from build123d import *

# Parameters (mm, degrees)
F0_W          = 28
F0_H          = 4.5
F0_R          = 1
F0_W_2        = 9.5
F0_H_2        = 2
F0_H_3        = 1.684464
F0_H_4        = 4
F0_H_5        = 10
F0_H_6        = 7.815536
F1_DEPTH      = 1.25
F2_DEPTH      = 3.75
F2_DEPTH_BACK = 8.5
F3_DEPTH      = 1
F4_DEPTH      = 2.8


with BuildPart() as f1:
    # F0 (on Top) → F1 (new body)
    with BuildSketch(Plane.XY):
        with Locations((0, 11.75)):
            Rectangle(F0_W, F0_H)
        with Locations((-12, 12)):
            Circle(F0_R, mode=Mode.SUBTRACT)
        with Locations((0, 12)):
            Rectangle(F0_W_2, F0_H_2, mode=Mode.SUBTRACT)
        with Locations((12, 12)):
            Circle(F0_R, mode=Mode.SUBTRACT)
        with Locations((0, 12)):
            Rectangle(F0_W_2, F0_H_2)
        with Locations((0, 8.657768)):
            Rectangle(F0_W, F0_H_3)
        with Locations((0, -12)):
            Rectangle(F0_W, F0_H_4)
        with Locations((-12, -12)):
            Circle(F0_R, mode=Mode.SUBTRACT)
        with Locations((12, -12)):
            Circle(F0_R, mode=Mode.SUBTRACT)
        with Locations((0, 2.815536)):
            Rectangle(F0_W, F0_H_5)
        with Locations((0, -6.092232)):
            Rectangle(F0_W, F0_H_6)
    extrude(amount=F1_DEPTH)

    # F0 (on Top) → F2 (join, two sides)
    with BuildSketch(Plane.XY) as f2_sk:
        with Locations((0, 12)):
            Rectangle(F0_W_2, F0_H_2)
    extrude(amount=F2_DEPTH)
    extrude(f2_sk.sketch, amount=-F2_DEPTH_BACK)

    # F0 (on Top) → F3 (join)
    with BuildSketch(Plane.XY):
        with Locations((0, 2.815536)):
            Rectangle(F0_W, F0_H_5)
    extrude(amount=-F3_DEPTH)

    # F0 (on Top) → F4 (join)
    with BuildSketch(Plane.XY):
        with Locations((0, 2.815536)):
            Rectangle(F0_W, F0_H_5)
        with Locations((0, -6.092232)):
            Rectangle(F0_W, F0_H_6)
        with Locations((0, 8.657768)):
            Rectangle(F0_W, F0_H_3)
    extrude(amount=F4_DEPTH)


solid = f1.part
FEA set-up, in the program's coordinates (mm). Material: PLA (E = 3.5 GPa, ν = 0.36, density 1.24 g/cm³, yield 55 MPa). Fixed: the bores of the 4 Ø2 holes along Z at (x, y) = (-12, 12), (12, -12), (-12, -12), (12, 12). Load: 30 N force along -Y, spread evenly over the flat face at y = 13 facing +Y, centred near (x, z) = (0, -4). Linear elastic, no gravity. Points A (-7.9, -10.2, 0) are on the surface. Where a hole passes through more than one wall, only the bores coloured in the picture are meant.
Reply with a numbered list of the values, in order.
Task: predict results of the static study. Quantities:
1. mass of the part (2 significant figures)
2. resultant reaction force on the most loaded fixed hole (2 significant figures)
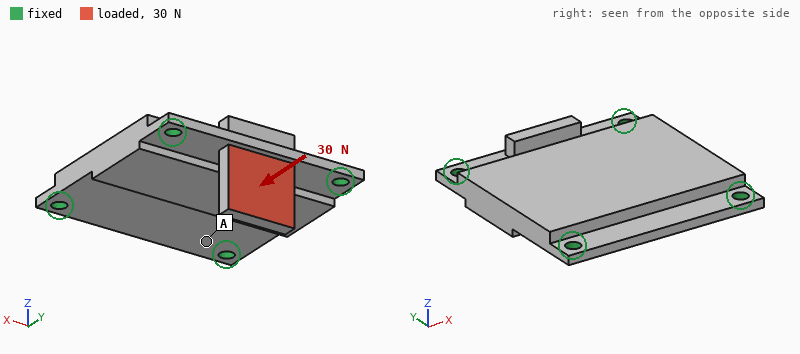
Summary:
1. 2.9 g
2. 12 N
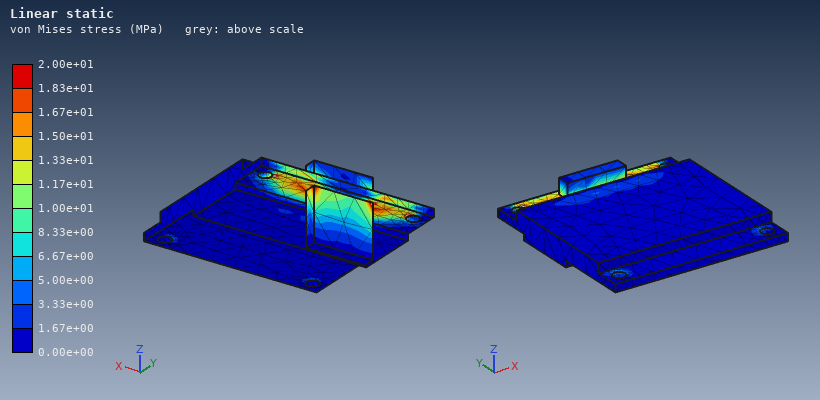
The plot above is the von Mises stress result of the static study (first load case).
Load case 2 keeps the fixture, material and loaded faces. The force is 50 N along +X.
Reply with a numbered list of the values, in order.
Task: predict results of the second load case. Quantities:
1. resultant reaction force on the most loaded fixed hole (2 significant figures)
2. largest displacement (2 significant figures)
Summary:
1. 24 N
2. 0.11 mm
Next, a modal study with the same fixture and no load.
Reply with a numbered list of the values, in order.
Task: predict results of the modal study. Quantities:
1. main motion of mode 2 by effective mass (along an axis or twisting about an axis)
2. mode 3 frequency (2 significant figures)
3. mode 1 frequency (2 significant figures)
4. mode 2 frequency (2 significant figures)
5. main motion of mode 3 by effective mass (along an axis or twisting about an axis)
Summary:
1. along Z
2. 6200 Hz
3. 3400 Hz
4. 3800 Hz
5. twisting about X
